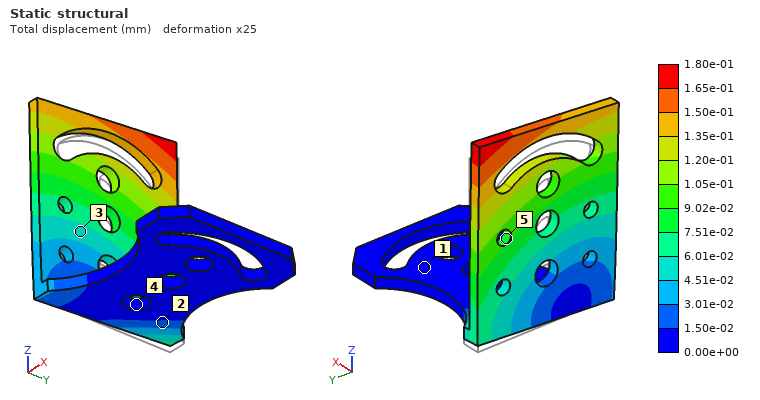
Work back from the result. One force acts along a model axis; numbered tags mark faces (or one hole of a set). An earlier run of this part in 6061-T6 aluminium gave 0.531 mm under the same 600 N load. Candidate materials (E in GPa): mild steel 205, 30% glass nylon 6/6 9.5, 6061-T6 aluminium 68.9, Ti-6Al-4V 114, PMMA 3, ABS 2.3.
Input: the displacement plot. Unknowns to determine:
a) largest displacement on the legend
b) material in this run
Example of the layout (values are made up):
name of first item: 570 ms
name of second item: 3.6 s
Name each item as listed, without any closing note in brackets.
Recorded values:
largest displacement on the legend: 1.80e-01 mm
material in this run: mild steel
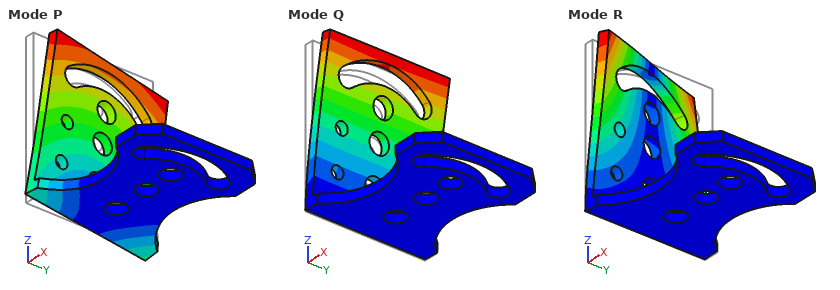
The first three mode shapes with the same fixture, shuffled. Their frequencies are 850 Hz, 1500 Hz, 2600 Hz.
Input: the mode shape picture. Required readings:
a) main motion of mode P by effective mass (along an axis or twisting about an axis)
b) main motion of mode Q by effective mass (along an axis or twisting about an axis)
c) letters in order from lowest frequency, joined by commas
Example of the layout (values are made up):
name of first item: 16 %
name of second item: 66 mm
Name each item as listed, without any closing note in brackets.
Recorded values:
main motion of mode P by effective mass: along Y
main motion of mode Q by effective mass: along X
letters in order from lowest frequency, joined by commas: Q, P, R
